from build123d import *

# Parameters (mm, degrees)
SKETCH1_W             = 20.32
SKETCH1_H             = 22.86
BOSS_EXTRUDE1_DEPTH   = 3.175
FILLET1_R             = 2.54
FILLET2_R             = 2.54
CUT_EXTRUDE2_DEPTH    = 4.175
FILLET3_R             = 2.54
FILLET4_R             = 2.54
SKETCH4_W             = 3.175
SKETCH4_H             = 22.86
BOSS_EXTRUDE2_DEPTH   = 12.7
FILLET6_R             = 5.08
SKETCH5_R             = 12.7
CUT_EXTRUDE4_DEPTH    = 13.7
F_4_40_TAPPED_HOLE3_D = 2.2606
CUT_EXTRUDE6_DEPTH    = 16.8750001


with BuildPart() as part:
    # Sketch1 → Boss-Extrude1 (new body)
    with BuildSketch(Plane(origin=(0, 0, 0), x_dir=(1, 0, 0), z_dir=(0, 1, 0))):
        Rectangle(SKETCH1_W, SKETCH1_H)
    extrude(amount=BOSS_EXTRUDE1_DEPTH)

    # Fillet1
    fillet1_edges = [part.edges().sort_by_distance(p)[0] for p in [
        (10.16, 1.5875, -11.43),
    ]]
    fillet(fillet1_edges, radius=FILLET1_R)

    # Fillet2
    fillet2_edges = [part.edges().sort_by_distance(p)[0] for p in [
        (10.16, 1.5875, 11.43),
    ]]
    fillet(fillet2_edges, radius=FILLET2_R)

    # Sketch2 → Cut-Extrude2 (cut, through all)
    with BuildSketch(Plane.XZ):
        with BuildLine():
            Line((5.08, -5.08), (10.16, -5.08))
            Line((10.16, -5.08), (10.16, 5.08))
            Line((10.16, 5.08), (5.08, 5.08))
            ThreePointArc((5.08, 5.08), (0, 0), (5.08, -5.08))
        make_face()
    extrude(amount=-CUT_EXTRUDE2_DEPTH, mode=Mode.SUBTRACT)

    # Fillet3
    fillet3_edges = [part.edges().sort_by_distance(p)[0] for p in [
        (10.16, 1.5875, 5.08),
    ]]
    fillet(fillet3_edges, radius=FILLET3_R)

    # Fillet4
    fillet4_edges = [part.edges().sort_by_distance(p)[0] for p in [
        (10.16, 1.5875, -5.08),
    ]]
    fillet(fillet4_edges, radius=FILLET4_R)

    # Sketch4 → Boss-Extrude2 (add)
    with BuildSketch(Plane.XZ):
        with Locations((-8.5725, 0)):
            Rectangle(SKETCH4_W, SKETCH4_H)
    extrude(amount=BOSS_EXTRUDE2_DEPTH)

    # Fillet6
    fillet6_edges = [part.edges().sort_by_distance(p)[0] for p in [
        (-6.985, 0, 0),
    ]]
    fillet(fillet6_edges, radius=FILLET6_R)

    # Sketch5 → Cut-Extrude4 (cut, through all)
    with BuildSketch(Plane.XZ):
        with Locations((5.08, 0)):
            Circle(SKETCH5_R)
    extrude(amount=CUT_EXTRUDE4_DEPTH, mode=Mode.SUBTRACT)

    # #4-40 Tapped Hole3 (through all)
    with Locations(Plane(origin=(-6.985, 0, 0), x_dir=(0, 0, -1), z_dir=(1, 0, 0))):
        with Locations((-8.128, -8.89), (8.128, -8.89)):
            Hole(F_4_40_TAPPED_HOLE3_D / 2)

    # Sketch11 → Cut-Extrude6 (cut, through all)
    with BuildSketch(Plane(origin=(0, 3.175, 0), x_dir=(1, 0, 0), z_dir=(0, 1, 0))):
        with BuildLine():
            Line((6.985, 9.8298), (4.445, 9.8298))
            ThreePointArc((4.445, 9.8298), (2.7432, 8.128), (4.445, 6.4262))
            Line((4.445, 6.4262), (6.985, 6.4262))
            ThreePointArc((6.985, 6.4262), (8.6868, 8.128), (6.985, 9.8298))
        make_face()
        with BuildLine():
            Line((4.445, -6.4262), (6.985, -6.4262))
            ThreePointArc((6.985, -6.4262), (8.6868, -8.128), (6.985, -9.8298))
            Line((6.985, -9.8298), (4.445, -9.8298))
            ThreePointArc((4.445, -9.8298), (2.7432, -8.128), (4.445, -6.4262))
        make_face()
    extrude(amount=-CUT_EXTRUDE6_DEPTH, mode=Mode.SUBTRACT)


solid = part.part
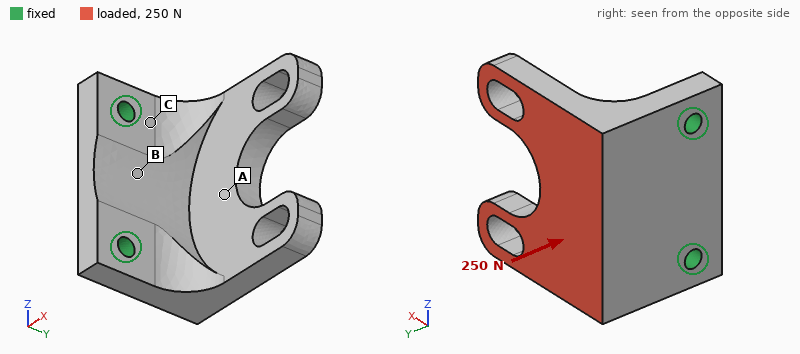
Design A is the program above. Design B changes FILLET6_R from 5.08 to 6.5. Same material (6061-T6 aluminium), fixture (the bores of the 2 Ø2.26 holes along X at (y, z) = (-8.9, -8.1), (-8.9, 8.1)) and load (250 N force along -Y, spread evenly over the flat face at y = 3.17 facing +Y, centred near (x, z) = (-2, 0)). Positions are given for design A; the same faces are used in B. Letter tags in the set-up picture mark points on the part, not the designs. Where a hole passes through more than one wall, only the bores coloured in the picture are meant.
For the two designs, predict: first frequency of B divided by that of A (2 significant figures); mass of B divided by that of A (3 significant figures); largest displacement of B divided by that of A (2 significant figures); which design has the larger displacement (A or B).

1.0
1.01
0.91
A
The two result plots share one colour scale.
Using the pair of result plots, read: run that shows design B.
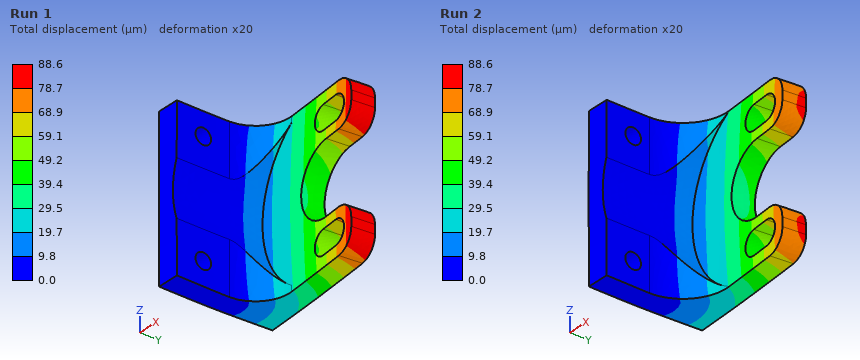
Run 2
